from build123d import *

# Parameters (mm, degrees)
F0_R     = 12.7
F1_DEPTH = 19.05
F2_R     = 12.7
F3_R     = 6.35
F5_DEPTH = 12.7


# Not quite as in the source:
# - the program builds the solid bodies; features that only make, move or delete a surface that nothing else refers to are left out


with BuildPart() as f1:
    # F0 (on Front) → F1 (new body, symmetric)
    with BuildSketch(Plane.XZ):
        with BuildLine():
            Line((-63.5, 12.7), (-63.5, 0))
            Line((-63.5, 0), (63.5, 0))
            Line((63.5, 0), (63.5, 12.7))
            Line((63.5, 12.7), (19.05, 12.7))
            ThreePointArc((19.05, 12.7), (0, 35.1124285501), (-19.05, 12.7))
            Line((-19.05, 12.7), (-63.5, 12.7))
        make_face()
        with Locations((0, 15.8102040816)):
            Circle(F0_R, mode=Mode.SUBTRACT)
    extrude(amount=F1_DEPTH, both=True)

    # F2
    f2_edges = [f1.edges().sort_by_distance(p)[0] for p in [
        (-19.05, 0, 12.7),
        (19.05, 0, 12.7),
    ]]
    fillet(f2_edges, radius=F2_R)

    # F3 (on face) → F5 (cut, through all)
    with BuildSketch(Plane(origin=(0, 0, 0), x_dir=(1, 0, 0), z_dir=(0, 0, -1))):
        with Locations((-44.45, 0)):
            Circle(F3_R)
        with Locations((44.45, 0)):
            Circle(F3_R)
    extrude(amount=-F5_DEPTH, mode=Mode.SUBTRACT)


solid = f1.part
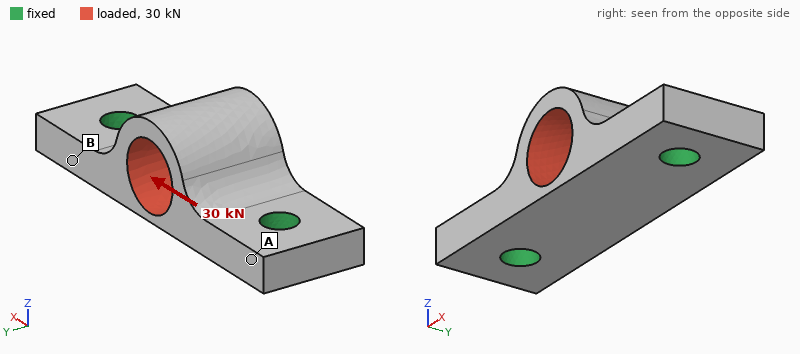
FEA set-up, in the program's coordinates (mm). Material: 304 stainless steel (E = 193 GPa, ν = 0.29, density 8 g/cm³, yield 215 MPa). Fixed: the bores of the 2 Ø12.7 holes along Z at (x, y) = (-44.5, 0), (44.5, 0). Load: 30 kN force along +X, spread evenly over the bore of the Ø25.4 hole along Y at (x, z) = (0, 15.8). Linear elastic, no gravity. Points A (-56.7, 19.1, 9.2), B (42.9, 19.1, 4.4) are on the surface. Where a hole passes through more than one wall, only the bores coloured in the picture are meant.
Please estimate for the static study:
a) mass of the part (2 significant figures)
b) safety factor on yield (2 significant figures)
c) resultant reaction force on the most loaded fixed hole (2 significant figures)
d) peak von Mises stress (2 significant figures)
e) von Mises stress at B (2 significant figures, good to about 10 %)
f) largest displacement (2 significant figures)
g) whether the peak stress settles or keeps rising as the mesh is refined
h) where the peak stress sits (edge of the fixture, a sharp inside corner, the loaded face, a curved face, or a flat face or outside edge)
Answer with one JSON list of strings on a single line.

["540 g", "2.2", "15 kN", "100 MPa", "15 MPa", "21 µm", "settles", "a curved face"]
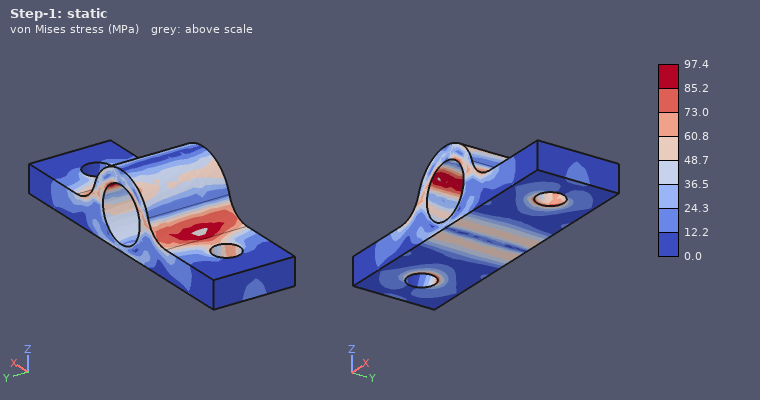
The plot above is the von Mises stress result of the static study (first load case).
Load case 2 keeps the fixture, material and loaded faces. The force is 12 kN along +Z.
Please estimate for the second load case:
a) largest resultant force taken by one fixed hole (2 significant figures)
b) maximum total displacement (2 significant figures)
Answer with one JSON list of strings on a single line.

["6.0 kN", "24 µm"]
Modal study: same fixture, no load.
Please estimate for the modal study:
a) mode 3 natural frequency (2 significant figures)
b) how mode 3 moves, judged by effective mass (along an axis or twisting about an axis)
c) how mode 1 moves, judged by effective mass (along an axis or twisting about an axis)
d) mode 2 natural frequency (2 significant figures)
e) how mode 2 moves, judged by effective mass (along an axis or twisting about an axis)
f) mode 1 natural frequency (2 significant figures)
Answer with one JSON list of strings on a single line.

["11 kHz", "along Y", "along Y", "8400 Hz", "along Z", "6800 Hz"]
